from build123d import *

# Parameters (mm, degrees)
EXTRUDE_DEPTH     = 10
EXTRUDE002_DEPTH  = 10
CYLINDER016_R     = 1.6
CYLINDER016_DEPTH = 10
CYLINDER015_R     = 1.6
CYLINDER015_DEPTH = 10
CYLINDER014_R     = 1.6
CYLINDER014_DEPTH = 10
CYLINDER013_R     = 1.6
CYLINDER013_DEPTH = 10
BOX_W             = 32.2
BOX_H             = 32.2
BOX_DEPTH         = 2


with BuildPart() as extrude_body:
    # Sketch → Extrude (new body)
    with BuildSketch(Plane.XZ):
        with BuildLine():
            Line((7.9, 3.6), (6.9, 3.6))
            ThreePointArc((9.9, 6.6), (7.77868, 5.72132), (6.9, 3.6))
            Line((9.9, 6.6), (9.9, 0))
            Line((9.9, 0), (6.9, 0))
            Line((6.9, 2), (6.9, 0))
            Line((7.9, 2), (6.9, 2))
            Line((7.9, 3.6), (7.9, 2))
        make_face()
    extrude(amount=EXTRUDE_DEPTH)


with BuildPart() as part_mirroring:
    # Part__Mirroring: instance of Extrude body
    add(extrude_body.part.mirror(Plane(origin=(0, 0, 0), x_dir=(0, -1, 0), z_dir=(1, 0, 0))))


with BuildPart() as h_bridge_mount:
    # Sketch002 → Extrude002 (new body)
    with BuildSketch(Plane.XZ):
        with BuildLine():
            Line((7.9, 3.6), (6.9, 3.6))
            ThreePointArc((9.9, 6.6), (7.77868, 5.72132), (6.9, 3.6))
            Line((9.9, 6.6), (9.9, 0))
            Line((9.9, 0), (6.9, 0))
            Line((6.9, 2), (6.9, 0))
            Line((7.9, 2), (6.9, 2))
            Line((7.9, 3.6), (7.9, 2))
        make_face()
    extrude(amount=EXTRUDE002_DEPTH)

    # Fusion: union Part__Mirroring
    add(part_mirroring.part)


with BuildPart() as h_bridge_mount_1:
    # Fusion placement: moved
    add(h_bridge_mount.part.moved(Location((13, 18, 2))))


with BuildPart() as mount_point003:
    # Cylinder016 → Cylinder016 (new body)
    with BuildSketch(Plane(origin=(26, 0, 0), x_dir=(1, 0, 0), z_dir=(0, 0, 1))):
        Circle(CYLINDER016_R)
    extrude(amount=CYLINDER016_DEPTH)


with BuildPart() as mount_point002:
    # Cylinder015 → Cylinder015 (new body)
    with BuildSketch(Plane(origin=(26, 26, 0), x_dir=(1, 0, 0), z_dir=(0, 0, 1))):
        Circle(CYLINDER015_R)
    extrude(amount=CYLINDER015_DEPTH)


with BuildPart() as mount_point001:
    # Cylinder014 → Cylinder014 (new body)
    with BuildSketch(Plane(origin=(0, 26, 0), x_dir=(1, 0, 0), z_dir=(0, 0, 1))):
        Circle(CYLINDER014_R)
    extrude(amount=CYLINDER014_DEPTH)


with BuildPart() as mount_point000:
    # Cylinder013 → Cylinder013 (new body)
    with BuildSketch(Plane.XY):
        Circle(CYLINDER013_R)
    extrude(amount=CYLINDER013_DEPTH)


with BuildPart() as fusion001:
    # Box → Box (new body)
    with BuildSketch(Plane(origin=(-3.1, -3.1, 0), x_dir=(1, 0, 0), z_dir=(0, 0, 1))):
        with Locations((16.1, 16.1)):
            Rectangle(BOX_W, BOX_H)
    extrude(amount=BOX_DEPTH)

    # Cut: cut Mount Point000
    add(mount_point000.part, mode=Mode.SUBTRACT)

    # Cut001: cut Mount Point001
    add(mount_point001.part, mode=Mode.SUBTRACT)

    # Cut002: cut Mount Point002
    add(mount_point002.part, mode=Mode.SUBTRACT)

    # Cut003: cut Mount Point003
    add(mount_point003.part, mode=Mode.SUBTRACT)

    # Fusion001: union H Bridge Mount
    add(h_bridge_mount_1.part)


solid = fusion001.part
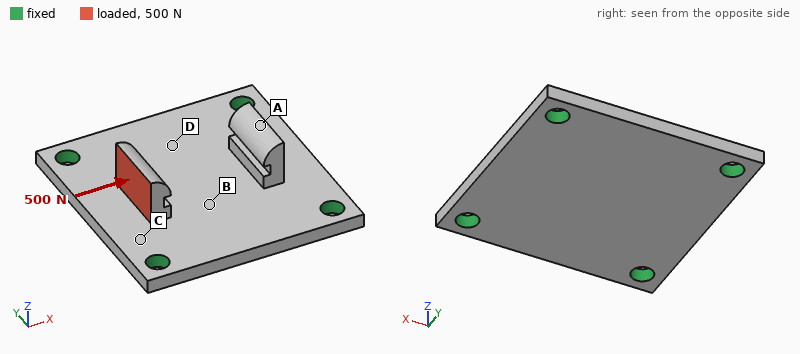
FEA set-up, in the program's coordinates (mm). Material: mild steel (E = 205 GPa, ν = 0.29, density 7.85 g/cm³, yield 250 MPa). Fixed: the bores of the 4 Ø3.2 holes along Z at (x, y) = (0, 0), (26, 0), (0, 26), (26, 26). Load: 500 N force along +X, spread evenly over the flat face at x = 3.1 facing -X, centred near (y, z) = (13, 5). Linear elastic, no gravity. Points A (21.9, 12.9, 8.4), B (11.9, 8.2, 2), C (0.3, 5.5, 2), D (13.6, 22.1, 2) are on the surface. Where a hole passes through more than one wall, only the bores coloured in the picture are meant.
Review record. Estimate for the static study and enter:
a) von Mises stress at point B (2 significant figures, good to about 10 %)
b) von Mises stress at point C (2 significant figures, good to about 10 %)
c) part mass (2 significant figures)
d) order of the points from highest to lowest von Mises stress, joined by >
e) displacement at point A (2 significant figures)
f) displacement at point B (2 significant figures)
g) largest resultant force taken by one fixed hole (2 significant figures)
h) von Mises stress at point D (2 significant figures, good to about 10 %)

37 MPa
50 MPa
18 g
C > B > D > A
4.8 µm
7.1 µm
160 N
22 MPa
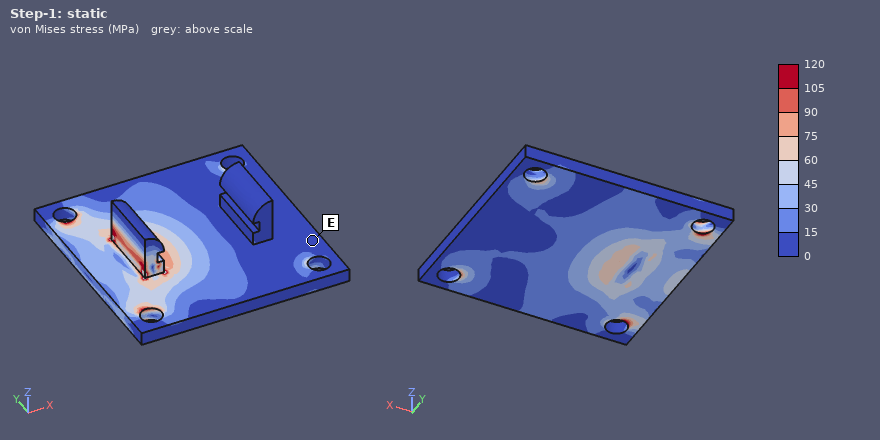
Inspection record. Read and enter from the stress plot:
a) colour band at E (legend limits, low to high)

0 to 15 MPa
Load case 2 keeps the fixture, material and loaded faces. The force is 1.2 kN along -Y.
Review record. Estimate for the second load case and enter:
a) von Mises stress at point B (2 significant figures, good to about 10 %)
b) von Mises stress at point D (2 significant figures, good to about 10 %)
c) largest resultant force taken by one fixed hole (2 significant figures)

40 MPa
18 MPa
540 N
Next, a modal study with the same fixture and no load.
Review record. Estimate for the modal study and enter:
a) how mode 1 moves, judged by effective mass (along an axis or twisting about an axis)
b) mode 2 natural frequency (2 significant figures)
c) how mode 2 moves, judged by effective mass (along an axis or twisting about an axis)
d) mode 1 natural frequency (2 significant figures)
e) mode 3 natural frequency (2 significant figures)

along Z
17 kHz
twisting about Y
11 kHz
19 kHz
